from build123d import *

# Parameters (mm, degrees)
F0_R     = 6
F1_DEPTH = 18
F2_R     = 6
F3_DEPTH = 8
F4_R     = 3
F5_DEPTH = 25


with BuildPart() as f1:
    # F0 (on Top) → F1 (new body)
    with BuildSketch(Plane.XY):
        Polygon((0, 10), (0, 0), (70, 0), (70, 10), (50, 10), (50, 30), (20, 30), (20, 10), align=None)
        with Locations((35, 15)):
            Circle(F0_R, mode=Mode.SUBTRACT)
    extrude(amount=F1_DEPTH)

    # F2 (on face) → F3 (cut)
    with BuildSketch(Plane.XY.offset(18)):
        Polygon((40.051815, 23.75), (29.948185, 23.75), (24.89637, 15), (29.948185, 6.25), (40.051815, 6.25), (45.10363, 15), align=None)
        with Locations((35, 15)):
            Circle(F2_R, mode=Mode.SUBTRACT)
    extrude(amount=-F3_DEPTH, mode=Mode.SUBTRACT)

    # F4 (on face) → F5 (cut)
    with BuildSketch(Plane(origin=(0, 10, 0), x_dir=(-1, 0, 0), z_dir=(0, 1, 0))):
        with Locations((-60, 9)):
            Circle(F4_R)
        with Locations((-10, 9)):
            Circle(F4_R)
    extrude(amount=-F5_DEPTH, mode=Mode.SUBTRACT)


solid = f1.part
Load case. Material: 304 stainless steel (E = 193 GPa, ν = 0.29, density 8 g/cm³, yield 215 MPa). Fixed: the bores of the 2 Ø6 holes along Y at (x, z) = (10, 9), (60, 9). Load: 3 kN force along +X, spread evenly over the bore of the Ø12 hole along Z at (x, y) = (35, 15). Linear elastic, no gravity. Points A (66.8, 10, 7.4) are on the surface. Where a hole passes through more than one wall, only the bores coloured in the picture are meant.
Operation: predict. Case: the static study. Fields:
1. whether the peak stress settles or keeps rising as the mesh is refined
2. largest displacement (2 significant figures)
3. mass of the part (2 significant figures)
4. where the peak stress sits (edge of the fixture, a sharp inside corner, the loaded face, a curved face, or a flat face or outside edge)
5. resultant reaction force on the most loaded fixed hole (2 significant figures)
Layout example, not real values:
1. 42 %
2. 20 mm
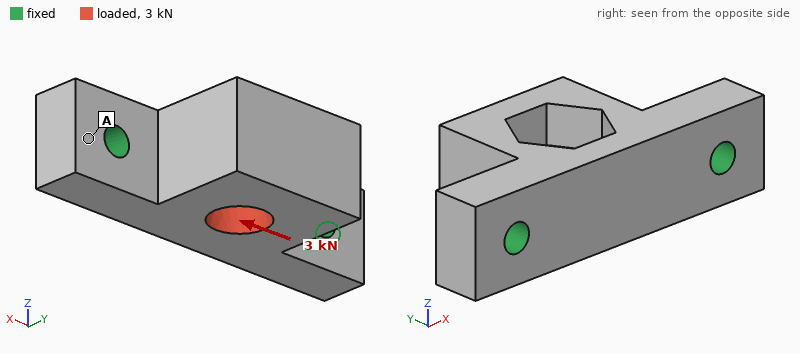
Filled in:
1. keeps rising
2. 4.3 µm
3. 160 g
4. edge of the fixture
5. 1.7 kN
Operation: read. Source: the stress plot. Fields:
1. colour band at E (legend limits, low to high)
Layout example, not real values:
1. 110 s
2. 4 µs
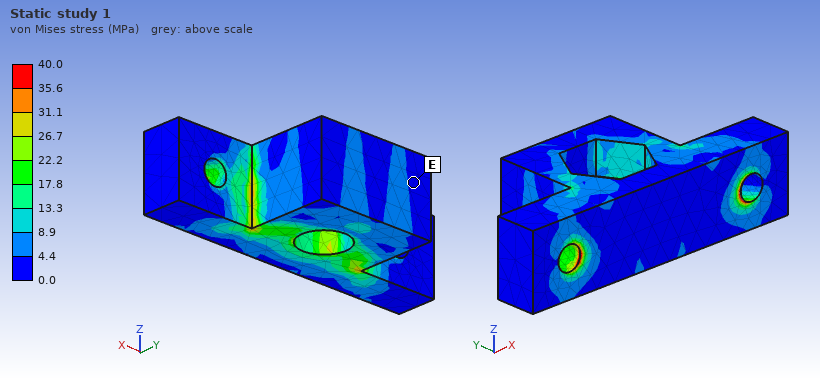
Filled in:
1. 0.0 to 4.4 MPa
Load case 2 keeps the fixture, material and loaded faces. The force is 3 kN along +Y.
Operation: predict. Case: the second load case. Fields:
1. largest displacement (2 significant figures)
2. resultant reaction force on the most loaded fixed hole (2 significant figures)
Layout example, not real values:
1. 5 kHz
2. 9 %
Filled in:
1. 9.0 µm
2. 1.5 kN
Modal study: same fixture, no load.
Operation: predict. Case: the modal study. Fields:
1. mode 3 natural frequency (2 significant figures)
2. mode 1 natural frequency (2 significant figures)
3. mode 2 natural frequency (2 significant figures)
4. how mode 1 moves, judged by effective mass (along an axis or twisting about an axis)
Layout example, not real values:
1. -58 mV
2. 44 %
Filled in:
1. 14 kHz
2. 6800 Hz
3. 14 kHz
4. along Z
